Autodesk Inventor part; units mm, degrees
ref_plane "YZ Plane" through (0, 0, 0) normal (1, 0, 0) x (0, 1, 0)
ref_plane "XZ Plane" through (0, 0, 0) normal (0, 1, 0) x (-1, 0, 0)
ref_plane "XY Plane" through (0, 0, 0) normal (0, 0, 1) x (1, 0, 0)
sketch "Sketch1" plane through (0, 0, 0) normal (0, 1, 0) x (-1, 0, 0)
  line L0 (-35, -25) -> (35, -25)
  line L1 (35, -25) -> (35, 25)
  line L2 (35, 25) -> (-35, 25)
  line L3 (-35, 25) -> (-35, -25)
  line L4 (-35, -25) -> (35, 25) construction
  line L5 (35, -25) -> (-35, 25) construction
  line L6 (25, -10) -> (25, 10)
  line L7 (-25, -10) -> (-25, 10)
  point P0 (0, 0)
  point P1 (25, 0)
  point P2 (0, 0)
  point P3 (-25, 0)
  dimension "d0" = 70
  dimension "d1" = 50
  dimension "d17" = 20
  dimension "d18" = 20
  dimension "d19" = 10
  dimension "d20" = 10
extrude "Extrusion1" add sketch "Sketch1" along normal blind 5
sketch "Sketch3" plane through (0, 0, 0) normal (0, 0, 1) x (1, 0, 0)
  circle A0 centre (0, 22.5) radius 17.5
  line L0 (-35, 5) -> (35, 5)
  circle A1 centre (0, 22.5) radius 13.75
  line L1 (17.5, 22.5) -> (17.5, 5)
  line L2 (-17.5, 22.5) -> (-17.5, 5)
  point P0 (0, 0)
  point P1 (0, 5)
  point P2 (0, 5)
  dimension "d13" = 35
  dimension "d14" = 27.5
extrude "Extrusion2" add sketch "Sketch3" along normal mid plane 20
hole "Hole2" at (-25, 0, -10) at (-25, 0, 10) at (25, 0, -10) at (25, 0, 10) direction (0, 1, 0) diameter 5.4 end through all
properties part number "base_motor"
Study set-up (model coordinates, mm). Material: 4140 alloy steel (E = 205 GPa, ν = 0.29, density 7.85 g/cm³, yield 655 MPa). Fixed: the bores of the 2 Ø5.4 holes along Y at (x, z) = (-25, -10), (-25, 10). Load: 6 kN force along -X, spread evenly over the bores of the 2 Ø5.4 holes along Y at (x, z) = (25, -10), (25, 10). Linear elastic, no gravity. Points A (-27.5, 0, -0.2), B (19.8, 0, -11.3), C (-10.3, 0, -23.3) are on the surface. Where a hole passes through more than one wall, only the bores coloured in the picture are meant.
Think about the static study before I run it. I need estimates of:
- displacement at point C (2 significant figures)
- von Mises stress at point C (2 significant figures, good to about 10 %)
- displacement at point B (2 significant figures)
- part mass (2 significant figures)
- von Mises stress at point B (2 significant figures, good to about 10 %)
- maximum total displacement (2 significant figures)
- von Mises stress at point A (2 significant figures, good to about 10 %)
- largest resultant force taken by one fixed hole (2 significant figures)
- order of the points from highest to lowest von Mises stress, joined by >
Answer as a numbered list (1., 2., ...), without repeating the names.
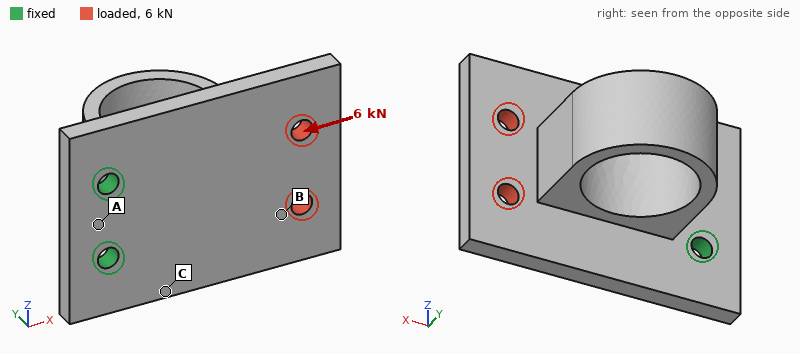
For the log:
1. 3.0 µm
2. 21 MPa
3. 12 µm
4. 210 g
5. 38 MPa
6. 20 µm
7. 10 MPa
8. 3.0 kN
9. B > C > A
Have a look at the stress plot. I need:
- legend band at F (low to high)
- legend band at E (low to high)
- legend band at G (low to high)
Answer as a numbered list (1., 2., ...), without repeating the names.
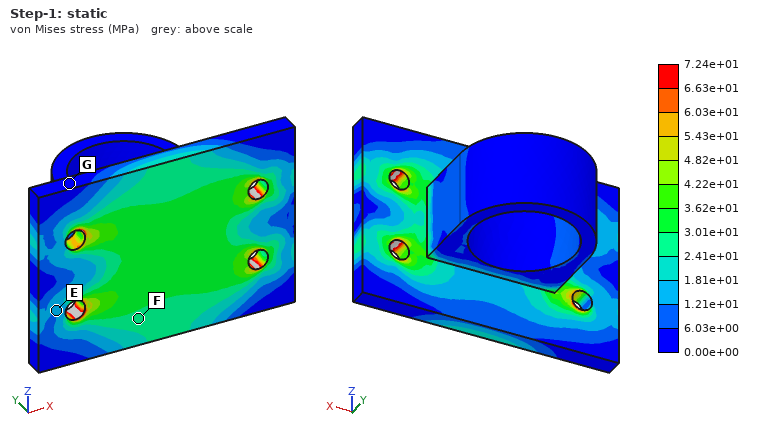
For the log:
1. 2.41e+01 to 3.01e+01 MPa
2. 1.21e+01 to 1.81e+01 MPa
3. 0.00e+00 to 6.03e+00 MPa
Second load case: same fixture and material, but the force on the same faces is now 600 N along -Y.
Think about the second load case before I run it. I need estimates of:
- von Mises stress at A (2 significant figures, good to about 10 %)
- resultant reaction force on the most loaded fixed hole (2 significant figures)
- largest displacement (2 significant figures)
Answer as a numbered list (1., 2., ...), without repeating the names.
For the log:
1. 27 MPa
2. 320 N
3. 0.19 mm
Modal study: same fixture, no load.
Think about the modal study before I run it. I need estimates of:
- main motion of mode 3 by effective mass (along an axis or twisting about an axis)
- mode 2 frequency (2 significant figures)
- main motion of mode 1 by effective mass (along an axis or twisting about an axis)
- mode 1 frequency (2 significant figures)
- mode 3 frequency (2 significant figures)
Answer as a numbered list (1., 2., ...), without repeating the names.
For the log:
1. along Z
2. 3500 Hz
3. along Y
4. 1100 Hz
5. 5600 Hz
